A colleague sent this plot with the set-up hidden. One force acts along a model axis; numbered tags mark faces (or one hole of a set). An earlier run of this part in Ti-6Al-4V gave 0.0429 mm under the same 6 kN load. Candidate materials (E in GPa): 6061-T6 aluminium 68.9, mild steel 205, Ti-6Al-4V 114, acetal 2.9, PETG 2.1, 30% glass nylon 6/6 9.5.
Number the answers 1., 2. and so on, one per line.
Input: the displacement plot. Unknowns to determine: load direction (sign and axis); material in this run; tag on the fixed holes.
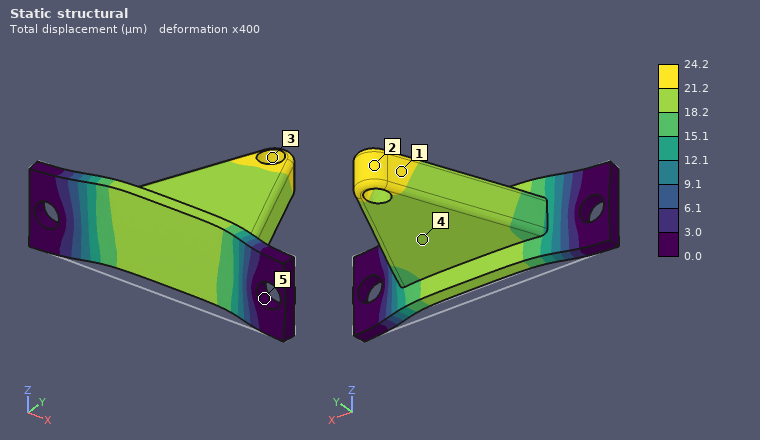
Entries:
1. +Y
2. mild steel
3. 5
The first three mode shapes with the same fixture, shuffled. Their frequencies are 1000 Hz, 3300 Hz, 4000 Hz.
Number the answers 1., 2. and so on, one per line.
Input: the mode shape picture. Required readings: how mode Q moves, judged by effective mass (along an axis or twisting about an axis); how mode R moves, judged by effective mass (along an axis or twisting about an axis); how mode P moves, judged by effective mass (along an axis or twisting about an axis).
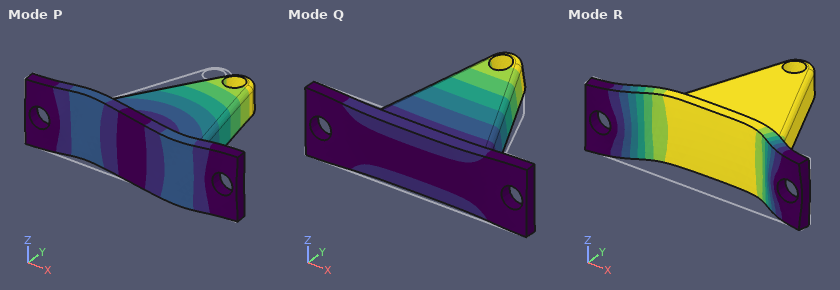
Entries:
1. along Z
2. along Y
3. along X
